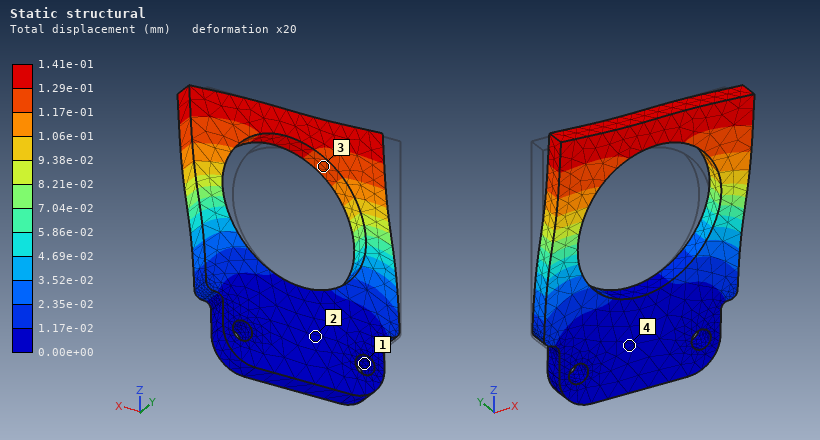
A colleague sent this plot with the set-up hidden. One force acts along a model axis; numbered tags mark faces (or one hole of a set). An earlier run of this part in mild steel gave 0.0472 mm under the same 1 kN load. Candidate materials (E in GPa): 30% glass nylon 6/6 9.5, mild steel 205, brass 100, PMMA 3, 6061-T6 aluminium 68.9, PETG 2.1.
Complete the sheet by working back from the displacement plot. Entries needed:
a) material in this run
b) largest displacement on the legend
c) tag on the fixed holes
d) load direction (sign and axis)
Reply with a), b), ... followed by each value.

a) 6061-T6 aluminium
b) 1.41e-01 mm
c) 1
d) +X
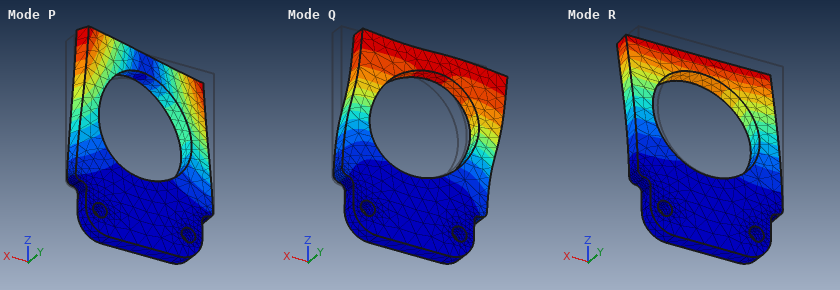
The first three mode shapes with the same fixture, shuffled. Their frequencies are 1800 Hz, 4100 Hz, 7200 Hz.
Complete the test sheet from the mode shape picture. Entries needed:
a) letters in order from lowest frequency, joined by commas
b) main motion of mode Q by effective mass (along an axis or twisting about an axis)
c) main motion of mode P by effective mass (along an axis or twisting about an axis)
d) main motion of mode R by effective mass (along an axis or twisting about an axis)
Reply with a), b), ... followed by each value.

a) R, P, Q
b) along X
c) twisting about Z
d) along Y
